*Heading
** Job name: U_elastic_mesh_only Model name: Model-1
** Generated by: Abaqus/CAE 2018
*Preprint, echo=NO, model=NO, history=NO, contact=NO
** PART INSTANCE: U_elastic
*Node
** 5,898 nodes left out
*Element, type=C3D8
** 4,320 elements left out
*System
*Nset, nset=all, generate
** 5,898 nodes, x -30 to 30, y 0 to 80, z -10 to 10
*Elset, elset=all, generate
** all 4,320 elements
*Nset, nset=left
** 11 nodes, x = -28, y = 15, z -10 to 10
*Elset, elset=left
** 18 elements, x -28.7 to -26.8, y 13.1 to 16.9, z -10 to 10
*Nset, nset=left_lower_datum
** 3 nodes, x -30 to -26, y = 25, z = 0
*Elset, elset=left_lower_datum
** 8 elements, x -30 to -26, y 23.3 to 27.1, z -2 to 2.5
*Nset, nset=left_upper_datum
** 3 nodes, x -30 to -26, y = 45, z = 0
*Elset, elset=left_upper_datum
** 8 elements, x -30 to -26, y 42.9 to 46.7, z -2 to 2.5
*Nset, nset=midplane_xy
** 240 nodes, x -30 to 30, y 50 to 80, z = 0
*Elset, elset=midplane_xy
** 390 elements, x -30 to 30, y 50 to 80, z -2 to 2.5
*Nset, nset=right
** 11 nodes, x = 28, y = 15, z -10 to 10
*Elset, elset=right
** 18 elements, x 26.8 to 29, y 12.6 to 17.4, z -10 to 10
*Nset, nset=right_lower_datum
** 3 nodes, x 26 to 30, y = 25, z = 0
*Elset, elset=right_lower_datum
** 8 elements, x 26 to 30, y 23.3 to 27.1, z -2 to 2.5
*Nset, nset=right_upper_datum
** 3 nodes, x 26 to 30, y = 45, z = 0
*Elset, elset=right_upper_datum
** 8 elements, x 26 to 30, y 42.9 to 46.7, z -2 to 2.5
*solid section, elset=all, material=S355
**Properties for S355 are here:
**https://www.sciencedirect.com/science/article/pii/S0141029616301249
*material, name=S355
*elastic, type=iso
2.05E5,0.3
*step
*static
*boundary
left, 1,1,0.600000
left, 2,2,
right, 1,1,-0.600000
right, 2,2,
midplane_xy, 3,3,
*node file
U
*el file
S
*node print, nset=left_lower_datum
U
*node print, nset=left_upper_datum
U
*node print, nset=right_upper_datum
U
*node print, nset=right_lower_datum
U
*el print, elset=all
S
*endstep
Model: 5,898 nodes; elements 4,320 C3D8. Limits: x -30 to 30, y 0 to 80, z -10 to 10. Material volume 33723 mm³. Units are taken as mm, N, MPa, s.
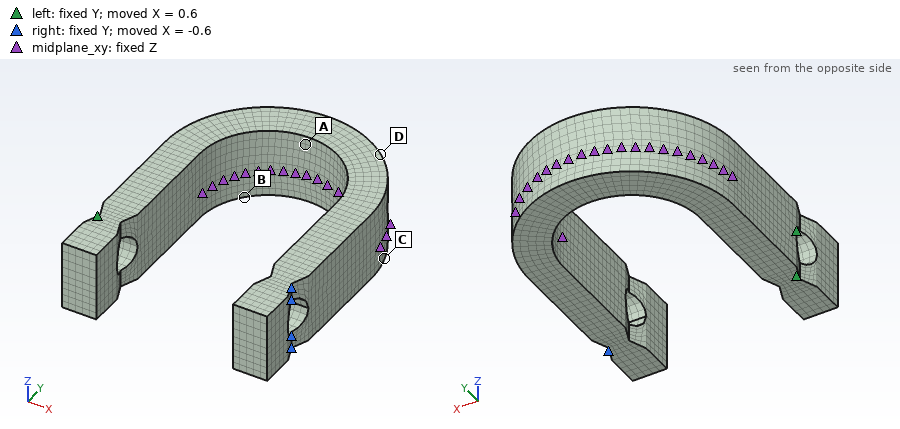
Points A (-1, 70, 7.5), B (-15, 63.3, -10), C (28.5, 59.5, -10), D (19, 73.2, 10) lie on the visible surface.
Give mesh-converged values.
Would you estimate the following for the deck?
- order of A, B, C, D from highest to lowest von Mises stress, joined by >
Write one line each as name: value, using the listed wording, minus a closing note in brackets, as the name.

order of A, B, C, D from highest to lowest von Mises stress, joined by >: A > B > D > C
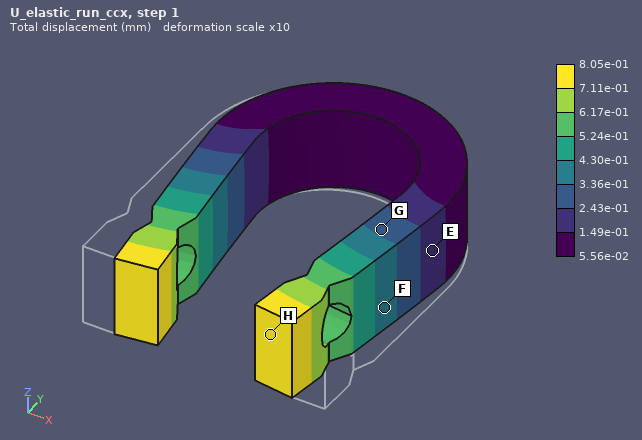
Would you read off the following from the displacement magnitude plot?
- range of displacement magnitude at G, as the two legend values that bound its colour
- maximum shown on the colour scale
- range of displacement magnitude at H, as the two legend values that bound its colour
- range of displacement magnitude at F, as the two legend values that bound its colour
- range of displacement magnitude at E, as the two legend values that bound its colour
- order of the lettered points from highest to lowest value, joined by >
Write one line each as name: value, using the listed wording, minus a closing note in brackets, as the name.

range of displacement magnitude at G, as the two legend values that bound its colour: 2.43e-01 to 3.36e-01 mm
maximum shown on the colour scale: 8.05e-01 mm
range of displacement magnitude at H, as the two legend values that bound its colour: 7.11e-01 to 8.05e-01 mm
range of displacement magnitude at F, as the two legend values that bound its colour: 3.36e-01 to 4.30e-01 mm
range of displacement magnitude at E, as the two legend values that bound its colour: 1.49e-01 to 2.43e-01 mm
order of the lettered points from highest to lowest value, joined by >: H > F > G > E
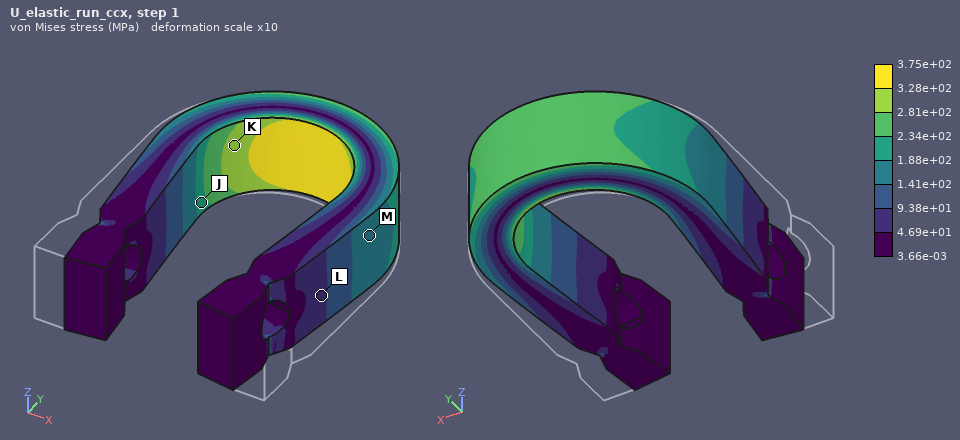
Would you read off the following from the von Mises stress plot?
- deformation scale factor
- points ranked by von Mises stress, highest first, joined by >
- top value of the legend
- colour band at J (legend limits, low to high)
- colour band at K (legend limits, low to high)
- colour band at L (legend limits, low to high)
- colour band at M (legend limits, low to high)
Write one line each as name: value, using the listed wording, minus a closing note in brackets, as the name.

deformation scale factor: 10
points ranked by von Mises stress, highest first, joined by >: K > J > M > L
top value of the legend: 3.75e+02 MPa
colour band at J: 1.88e+02 to 2.34e+02 MPa
colour band at K: 2.81e+02 to 3.28e+02 MPa
colour band at L: 4.69e+01 to 9.38e+01 MPa
colour band at M: 1.41e+02 to 1.88e+02 MPa
